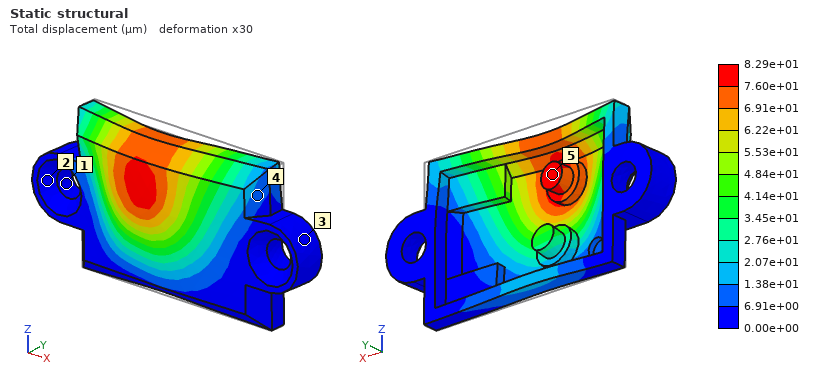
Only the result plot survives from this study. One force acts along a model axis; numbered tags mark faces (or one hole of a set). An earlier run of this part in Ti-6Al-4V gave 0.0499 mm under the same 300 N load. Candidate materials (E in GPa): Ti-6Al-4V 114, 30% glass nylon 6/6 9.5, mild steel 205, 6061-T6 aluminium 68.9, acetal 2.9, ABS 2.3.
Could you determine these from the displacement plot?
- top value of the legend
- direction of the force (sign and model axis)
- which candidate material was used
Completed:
8.29e+01 µm
-Y
6061-T6 aluminium
